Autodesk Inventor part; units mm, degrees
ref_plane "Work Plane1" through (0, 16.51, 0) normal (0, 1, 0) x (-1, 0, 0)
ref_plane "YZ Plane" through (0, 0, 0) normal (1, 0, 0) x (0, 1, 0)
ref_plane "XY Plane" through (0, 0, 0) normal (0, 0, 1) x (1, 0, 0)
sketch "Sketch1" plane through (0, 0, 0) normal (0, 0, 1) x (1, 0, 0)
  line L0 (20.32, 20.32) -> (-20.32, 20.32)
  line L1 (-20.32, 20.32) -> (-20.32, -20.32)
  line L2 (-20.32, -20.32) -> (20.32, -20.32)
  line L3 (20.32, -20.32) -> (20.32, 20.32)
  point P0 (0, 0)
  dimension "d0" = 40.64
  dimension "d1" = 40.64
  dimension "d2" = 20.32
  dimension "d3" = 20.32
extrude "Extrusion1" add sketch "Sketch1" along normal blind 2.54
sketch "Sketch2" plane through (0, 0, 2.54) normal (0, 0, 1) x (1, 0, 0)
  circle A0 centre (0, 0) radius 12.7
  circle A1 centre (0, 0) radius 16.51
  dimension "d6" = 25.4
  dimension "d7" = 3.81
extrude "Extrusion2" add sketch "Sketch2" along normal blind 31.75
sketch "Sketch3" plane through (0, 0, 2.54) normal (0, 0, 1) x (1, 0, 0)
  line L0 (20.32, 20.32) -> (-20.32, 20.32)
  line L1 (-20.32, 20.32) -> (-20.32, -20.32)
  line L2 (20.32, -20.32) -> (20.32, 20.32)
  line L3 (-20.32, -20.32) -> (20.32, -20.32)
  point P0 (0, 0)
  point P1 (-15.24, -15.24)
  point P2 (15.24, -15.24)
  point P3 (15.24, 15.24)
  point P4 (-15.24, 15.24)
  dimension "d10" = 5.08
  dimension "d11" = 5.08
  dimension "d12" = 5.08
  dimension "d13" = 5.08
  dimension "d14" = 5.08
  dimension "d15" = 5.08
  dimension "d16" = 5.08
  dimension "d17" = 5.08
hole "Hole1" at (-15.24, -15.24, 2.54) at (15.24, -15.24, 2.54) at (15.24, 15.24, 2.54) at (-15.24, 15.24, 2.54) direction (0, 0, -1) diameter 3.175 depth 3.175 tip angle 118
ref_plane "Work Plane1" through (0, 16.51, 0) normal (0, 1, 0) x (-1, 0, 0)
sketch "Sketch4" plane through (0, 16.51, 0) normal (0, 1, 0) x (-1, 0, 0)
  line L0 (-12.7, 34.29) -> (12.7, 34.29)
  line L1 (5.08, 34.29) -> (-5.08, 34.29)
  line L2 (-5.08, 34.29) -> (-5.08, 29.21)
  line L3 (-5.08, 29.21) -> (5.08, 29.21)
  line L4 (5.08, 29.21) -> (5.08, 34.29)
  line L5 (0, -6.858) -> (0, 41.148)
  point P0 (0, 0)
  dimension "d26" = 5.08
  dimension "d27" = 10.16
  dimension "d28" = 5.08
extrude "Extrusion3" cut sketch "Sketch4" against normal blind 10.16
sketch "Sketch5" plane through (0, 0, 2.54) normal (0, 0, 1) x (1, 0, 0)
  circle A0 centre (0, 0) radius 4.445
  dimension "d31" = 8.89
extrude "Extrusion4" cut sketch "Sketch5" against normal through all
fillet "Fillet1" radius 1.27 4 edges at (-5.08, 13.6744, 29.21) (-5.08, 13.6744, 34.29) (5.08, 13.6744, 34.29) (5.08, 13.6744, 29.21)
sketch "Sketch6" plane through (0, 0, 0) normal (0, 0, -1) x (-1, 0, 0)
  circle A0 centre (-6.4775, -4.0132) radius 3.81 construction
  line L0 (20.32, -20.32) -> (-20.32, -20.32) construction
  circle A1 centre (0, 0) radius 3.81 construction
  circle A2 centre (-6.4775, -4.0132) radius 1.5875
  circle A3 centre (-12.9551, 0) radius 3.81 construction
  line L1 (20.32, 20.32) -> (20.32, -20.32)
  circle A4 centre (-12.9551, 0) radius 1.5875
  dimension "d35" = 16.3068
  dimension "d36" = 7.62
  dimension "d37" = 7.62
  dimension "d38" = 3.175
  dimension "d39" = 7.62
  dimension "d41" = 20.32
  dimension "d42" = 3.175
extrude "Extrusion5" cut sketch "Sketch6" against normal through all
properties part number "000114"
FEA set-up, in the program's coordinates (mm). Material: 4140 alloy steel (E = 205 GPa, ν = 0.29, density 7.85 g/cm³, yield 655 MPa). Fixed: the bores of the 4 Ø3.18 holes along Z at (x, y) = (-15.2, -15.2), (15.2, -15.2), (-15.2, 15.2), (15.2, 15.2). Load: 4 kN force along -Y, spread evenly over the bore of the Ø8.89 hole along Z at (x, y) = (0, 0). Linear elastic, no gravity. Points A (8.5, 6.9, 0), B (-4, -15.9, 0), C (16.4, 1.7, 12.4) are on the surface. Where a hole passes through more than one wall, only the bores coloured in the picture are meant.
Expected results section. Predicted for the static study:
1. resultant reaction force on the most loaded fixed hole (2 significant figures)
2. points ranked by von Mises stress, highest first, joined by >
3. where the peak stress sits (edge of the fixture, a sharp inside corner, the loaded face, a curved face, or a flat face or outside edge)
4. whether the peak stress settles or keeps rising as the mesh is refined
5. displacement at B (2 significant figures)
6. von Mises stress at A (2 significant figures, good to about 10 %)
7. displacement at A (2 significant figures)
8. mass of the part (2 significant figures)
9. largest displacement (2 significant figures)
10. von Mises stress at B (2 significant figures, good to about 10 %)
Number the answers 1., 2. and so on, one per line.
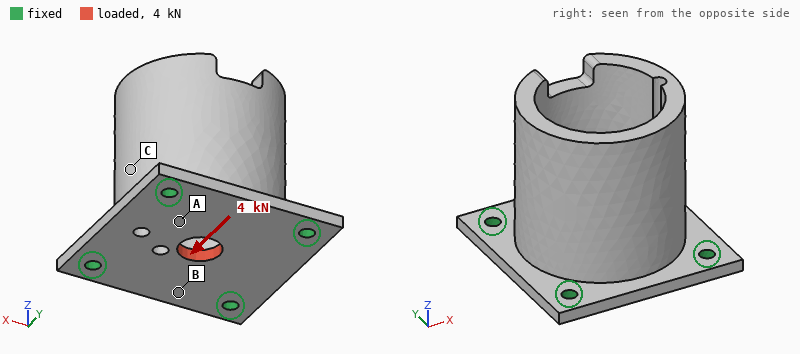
1. 1.1 kN
2. A > B > C
3. edge of the fixture
4. keeps rising
5. 3.1 µm
6. 38 MPa
7. 2.5 µm
8. 120 g
9. 5.2 µm
10. 20 MPa
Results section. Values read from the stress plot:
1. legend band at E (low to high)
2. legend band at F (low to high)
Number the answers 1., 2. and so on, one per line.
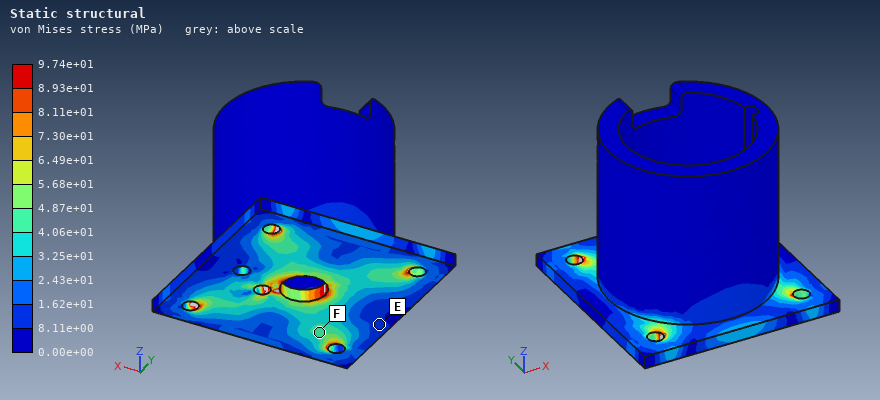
1. 8.11e+00 to 1.62e+01 MPa
2. 4.06e+01 to 4.87e+01 MPa
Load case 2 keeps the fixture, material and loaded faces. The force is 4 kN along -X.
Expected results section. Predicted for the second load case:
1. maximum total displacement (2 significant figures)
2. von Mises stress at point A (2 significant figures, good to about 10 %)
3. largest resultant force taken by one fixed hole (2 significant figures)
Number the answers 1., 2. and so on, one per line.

1. 5.7 µm
2. 36 MPa
3. 1.1 kN
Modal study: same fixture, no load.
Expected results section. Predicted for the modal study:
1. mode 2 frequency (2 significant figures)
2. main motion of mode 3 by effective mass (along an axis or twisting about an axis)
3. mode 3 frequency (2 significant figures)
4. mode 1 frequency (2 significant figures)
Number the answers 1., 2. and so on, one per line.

1. 6300 Hz
2. along Z
3. 9800 Hz
4. 6300 Hz
